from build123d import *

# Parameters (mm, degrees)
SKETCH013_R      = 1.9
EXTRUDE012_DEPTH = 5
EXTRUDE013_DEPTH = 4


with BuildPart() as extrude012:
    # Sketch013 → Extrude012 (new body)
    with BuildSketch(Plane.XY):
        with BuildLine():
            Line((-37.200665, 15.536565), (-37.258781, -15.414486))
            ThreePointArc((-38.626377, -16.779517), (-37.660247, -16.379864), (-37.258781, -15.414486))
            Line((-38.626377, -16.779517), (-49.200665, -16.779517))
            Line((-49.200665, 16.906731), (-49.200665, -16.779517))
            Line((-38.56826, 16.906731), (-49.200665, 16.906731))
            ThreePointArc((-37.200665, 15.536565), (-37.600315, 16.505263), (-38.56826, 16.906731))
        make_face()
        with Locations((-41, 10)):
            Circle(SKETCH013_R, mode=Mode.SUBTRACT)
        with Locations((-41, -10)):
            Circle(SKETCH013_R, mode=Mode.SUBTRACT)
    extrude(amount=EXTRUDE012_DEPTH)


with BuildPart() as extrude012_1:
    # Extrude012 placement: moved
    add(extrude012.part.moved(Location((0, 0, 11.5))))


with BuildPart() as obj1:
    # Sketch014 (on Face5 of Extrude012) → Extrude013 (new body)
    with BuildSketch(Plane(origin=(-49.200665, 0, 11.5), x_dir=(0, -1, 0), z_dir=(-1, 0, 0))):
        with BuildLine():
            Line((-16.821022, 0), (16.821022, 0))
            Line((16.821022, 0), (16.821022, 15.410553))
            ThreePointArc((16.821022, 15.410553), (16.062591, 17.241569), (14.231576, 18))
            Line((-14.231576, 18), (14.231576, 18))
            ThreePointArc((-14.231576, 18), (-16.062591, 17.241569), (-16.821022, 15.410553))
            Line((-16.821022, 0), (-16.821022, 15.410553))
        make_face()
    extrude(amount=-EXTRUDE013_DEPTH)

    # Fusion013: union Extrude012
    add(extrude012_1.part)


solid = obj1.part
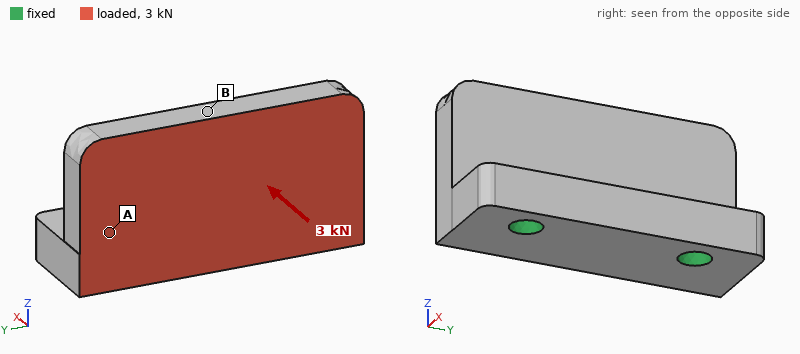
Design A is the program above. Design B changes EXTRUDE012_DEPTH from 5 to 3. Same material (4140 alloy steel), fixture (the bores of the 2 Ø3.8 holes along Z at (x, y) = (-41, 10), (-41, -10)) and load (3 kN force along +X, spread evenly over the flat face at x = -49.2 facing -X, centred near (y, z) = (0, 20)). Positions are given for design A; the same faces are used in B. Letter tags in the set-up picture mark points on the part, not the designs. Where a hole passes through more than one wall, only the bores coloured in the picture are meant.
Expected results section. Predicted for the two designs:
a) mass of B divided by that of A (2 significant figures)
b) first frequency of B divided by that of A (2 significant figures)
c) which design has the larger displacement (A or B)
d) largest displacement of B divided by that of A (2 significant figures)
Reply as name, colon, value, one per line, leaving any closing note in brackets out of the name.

mass of B divided by that of A: 0.87
first frequency of B divided by that of A: 0.55
which design has the larger displacement: B
largest displacement of B divided by that of A: 3.2
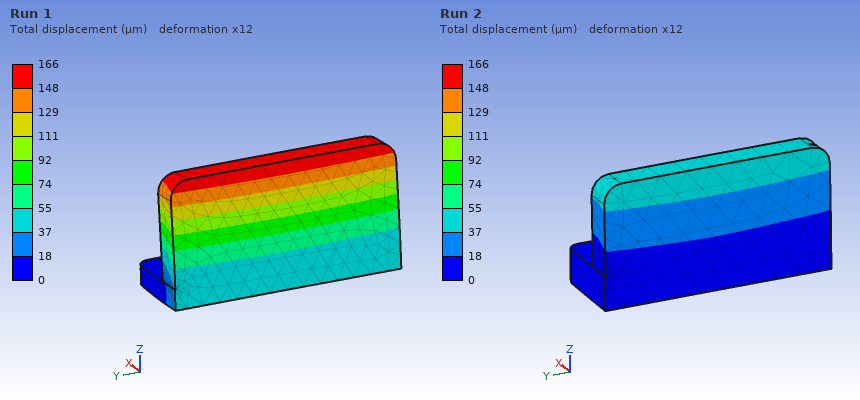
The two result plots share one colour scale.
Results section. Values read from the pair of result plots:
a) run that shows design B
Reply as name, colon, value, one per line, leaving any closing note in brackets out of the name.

run that shows design B: Run 1
